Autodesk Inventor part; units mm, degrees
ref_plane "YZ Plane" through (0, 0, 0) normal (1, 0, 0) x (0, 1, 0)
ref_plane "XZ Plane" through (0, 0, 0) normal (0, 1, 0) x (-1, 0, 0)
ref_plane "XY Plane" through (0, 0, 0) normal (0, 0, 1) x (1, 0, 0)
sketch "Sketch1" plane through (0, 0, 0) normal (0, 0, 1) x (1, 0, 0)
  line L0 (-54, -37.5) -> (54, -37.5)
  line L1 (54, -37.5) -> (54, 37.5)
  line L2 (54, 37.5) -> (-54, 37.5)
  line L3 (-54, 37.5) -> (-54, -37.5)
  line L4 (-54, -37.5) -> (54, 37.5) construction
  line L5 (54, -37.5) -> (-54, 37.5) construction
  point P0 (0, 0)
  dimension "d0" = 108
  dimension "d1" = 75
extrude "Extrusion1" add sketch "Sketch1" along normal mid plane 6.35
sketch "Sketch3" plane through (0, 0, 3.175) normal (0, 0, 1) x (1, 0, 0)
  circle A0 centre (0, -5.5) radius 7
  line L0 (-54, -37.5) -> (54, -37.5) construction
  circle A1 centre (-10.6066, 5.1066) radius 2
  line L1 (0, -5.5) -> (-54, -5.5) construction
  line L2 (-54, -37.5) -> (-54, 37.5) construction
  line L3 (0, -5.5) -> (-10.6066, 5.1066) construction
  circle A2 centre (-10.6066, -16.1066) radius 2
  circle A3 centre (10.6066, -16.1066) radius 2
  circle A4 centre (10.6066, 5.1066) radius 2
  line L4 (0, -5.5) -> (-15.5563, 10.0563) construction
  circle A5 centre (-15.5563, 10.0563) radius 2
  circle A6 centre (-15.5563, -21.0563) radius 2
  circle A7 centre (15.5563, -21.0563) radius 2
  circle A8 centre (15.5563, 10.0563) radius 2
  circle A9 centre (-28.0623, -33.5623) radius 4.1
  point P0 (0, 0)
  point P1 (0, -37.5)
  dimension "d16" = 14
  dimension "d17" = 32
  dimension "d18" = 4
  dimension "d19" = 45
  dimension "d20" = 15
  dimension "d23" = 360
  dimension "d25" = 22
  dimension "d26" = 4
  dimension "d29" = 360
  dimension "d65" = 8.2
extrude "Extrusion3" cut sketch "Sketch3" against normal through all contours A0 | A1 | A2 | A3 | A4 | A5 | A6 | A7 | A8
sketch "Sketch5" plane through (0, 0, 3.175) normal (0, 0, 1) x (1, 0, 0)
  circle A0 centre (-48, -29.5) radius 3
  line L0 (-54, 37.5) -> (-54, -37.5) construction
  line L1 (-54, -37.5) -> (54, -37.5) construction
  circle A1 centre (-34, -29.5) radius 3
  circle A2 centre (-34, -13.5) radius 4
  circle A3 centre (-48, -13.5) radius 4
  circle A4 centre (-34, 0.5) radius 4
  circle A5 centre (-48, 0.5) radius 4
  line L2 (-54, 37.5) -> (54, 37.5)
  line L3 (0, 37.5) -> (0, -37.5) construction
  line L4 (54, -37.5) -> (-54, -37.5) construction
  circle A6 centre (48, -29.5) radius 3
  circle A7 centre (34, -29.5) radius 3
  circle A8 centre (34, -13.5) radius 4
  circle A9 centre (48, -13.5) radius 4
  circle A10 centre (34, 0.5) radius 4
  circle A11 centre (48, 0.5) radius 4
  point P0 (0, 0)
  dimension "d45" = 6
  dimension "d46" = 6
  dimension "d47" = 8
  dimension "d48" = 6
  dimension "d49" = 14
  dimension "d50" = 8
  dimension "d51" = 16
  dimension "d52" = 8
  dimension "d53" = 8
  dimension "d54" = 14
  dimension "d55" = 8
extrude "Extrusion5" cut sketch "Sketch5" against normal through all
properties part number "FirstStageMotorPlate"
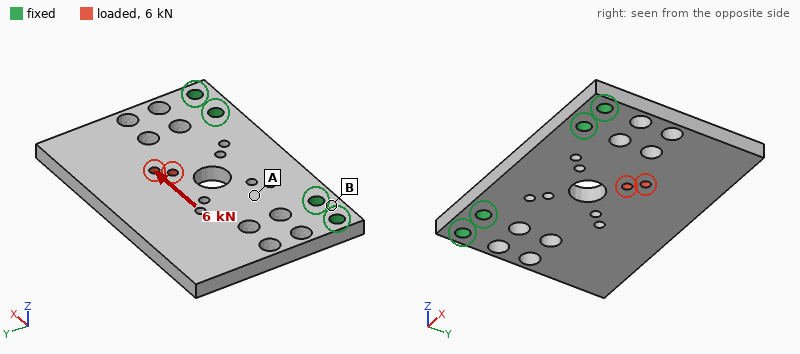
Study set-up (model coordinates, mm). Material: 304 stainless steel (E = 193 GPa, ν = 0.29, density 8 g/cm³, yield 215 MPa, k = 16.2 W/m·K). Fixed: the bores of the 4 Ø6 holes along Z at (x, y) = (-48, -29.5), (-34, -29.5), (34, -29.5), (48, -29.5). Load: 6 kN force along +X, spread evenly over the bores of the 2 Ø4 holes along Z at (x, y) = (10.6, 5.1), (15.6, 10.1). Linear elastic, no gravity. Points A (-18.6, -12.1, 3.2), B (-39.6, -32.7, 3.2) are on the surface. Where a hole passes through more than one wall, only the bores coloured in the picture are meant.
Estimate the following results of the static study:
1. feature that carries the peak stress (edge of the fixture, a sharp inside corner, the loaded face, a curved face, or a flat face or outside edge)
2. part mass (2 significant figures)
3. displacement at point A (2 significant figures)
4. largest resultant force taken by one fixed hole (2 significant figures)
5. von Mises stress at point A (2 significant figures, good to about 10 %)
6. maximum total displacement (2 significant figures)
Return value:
the loaded face
370 g
3.3 µm
2.4 kN
22 MPa
12 µm
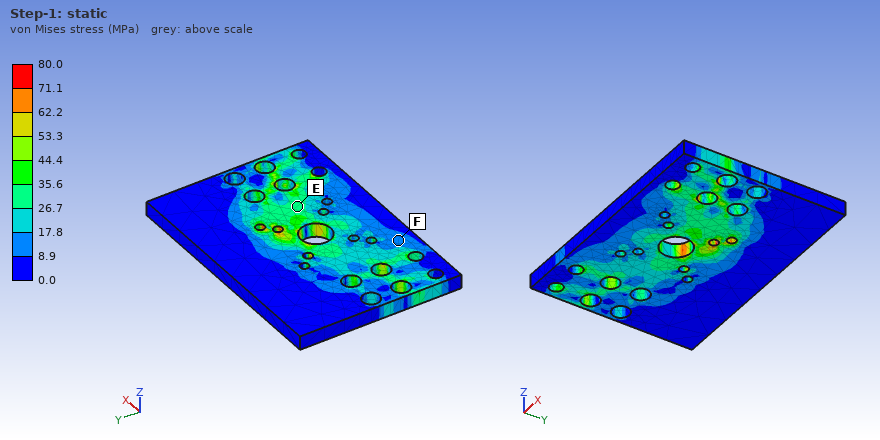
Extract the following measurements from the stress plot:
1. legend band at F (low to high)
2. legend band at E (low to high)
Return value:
8.9 to 17.8 MPa
26.7 to 35.6 MPa
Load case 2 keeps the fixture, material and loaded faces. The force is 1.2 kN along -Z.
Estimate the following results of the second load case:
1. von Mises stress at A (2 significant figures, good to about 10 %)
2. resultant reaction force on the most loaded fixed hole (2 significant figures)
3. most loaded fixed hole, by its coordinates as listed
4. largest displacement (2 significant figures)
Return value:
39 MPa
860 N
(34, -29.5)
0.19 mm
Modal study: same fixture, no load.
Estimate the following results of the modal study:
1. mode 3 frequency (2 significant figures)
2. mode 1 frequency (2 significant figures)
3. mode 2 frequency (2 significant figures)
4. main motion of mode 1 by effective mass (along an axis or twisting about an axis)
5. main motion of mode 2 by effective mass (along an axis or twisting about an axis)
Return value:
3800 Hz
900 Hz
1800 Hz
along Z
twisting about Y
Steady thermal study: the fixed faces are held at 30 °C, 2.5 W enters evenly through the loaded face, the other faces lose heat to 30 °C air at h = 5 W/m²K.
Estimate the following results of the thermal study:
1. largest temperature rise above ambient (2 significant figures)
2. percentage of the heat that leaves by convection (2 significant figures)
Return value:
19 K
26 %
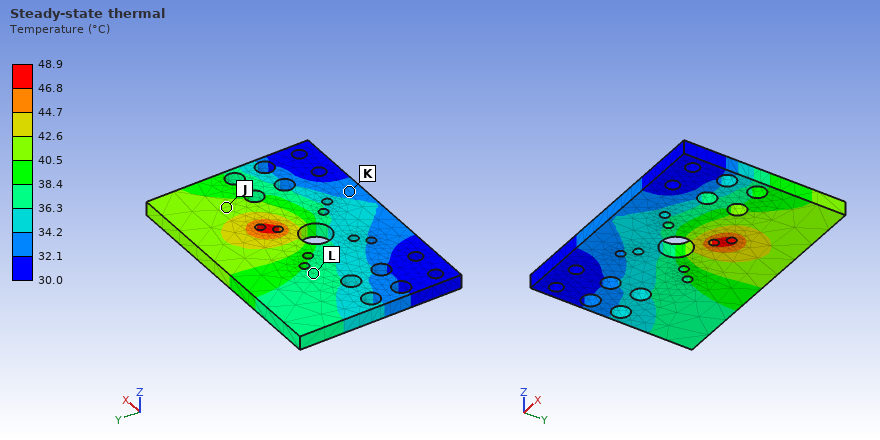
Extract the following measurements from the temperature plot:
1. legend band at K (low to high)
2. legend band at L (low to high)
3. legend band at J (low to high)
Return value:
32.1 to 34.2 °C
36.3 to 38.4 °C
40.5 to 42.6 °C
